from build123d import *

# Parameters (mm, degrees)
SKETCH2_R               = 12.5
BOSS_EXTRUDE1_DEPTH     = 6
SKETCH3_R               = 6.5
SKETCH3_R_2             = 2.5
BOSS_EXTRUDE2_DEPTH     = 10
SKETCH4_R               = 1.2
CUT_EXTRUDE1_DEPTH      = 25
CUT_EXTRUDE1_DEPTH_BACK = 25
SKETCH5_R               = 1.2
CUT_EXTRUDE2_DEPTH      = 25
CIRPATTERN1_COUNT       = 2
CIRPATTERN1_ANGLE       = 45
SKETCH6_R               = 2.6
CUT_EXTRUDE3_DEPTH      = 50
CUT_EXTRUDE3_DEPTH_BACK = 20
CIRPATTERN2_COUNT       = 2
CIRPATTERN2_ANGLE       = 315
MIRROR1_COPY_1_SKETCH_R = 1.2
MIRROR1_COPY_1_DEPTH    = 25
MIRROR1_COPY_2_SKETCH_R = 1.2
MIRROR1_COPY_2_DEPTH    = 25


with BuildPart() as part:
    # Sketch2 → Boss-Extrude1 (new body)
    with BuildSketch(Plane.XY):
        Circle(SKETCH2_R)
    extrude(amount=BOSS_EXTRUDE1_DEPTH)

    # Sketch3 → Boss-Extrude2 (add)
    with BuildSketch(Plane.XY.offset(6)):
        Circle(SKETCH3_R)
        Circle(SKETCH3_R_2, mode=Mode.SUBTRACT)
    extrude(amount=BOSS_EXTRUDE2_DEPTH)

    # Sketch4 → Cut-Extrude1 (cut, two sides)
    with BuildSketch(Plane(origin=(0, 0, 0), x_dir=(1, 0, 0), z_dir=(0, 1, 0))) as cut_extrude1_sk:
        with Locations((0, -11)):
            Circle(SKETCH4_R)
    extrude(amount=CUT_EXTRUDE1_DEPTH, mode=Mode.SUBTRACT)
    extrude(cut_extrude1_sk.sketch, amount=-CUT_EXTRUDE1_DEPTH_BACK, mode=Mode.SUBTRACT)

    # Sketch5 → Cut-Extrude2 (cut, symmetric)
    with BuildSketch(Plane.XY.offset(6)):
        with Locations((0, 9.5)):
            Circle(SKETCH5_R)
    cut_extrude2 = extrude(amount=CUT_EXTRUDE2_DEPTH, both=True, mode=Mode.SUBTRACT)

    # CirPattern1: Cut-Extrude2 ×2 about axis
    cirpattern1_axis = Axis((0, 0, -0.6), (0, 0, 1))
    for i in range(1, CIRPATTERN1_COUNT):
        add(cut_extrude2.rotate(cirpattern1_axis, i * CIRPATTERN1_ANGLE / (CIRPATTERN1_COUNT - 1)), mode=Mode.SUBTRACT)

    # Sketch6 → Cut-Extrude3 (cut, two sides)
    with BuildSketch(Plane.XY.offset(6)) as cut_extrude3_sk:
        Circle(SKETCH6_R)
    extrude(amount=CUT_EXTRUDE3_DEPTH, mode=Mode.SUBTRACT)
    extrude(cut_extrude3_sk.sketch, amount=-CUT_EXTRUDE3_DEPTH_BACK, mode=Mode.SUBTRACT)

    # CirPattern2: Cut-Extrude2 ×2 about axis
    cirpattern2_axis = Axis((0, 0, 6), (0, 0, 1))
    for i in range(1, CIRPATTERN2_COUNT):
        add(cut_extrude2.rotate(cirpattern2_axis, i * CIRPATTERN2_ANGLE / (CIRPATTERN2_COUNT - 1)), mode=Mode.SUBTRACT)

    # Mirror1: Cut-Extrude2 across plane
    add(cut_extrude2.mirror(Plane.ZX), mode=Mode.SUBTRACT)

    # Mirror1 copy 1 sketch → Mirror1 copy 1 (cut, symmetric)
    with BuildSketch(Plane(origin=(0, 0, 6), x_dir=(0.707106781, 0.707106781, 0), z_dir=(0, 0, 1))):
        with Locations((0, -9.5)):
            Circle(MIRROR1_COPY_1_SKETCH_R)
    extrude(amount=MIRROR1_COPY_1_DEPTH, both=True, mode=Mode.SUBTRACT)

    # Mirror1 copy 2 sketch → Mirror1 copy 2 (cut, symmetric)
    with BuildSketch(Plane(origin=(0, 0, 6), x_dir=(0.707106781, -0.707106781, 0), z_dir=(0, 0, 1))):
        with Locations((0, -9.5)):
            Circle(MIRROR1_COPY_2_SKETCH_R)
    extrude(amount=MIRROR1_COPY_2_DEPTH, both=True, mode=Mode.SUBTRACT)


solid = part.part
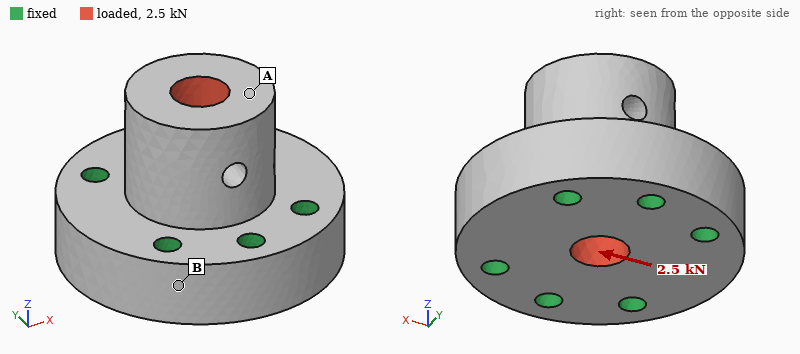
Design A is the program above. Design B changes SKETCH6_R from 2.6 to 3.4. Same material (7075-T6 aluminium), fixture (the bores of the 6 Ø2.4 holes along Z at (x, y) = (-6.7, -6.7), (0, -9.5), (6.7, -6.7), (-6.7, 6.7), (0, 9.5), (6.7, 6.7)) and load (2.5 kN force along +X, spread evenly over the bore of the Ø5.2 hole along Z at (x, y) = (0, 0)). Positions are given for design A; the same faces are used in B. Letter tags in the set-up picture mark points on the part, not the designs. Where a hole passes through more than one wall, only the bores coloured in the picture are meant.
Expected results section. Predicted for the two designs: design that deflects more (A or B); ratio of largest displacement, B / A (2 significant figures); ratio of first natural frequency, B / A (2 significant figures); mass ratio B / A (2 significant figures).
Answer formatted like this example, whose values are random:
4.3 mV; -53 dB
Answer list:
B; 1.1; 1.0; 0.94
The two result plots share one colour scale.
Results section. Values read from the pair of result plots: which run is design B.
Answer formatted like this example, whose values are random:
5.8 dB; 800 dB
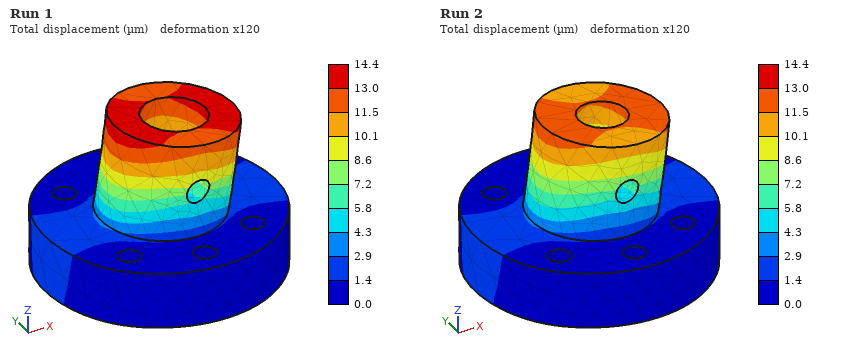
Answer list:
Run 1
